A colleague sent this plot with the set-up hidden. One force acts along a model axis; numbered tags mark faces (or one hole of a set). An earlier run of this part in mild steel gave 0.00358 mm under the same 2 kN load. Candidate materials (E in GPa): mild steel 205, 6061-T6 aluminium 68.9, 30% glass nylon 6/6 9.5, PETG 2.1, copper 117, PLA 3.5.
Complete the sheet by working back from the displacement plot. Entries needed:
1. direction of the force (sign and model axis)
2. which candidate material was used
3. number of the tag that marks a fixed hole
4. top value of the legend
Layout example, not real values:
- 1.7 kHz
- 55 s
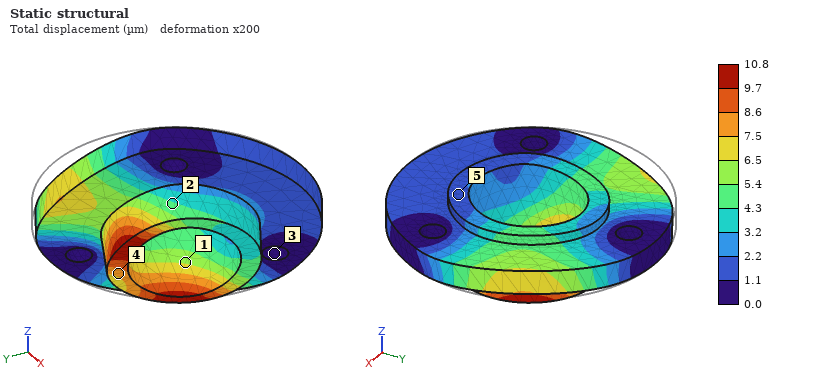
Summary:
- +X
- 6061-T6 aluminium
- 3
- 10.8 µm
